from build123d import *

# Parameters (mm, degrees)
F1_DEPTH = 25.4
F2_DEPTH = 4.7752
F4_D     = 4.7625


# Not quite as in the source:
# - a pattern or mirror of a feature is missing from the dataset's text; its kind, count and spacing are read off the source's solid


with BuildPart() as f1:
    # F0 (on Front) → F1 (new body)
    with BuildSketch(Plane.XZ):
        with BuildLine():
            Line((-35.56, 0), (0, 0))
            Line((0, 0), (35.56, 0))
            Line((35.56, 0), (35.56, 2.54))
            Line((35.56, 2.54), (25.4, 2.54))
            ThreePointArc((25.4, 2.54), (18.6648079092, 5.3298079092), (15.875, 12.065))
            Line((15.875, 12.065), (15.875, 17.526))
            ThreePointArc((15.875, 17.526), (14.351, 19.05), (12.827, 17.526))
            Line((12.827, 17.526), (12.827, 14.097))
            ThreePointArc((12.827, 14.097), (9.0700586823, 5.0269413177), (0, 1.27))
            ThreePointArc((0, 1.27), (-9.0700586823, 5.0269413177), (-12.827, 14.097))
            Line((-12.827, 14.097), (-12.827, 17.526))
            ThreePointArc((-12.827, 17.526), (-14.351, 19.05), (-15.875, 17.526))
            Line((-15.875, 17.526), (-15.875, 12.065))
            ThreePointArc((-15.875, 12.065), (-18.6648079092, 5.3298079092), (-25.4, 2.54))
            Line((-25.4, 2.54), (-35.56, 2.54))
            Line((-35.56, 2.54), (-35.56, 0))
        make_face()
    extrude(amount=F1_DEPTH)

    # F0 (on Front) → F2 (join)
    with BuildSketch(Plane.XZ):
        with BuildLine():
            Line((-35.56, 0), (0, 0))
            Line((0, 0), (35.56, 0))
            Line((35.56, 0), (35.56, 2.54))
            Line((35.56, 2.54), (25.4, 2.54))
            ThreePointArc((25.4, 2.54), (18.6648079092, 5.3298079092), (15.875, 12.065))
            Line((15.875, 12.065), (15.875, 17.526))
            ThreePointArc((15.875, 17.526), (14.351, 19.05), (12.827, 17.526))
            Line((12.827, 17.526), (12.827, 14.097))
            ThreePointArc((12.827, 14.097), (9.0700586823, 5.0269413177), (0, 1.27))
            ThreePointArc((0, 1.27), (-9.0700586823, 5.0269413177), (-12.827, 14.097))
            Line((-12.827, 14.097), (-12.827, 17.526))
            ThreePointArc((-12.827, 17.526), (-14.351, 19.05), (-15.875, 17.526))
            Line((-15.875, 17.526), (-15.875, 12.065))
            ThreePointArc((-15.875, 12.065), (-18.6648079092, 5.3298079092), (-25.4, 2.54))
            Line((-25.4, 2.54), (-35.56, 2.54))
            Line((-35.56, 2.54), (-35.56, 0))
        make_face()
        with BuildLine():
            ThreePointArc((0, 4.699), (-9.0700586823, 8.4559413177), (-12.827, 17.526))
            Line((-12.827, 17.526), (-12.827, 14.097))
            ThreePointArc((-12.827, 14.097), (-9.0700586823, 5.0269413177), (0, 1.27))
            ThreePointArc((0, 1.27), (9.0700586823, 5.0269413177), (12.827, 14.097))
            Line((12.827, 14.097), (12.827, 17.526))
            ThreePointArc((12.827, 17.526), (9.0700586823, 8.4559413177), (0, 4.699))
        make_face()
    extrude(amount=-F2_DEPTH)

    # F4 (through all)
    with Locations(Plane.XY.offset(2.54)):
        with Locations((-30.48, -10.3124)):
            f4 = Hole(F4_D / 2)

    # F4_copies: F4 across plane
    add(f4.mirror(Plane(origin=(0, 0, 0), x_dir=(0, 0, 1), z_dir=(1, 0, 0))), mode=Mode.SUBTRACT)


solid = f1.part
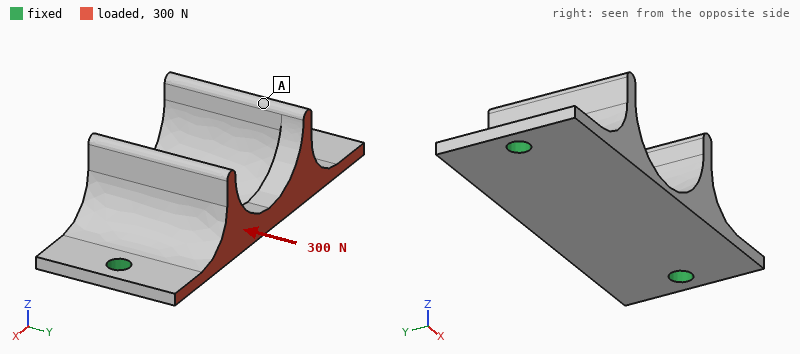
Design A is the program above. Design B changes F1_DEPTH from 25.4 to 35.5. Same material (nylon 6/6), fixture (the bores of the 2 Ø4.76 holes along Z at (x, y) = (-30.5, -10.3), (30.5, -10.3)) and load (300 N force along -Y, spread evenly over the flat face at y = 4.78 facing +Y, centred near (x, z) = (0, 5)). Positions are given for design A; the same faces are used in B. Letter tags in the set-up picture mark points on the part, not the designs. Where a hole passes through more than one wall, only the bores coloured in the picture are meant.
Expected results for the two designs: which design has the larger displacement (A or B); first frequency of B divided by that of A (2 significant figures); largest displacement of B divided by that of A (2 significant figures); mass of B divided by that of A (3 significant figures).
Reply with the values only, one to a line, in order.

B
0.69
1.1
1.32
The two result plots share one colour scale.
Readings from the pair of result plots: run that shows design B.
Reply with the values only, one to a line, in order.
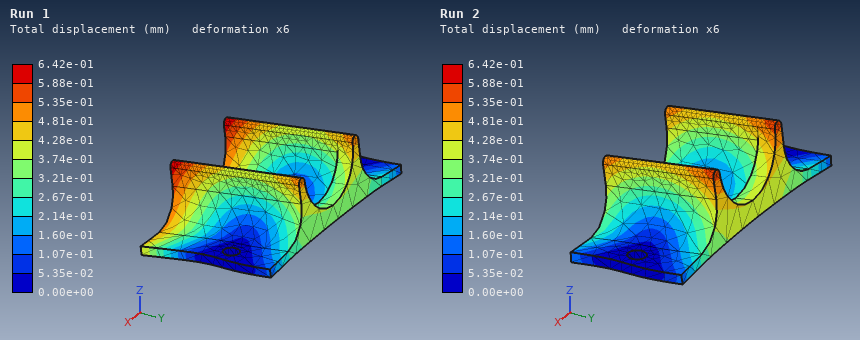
Run 1
